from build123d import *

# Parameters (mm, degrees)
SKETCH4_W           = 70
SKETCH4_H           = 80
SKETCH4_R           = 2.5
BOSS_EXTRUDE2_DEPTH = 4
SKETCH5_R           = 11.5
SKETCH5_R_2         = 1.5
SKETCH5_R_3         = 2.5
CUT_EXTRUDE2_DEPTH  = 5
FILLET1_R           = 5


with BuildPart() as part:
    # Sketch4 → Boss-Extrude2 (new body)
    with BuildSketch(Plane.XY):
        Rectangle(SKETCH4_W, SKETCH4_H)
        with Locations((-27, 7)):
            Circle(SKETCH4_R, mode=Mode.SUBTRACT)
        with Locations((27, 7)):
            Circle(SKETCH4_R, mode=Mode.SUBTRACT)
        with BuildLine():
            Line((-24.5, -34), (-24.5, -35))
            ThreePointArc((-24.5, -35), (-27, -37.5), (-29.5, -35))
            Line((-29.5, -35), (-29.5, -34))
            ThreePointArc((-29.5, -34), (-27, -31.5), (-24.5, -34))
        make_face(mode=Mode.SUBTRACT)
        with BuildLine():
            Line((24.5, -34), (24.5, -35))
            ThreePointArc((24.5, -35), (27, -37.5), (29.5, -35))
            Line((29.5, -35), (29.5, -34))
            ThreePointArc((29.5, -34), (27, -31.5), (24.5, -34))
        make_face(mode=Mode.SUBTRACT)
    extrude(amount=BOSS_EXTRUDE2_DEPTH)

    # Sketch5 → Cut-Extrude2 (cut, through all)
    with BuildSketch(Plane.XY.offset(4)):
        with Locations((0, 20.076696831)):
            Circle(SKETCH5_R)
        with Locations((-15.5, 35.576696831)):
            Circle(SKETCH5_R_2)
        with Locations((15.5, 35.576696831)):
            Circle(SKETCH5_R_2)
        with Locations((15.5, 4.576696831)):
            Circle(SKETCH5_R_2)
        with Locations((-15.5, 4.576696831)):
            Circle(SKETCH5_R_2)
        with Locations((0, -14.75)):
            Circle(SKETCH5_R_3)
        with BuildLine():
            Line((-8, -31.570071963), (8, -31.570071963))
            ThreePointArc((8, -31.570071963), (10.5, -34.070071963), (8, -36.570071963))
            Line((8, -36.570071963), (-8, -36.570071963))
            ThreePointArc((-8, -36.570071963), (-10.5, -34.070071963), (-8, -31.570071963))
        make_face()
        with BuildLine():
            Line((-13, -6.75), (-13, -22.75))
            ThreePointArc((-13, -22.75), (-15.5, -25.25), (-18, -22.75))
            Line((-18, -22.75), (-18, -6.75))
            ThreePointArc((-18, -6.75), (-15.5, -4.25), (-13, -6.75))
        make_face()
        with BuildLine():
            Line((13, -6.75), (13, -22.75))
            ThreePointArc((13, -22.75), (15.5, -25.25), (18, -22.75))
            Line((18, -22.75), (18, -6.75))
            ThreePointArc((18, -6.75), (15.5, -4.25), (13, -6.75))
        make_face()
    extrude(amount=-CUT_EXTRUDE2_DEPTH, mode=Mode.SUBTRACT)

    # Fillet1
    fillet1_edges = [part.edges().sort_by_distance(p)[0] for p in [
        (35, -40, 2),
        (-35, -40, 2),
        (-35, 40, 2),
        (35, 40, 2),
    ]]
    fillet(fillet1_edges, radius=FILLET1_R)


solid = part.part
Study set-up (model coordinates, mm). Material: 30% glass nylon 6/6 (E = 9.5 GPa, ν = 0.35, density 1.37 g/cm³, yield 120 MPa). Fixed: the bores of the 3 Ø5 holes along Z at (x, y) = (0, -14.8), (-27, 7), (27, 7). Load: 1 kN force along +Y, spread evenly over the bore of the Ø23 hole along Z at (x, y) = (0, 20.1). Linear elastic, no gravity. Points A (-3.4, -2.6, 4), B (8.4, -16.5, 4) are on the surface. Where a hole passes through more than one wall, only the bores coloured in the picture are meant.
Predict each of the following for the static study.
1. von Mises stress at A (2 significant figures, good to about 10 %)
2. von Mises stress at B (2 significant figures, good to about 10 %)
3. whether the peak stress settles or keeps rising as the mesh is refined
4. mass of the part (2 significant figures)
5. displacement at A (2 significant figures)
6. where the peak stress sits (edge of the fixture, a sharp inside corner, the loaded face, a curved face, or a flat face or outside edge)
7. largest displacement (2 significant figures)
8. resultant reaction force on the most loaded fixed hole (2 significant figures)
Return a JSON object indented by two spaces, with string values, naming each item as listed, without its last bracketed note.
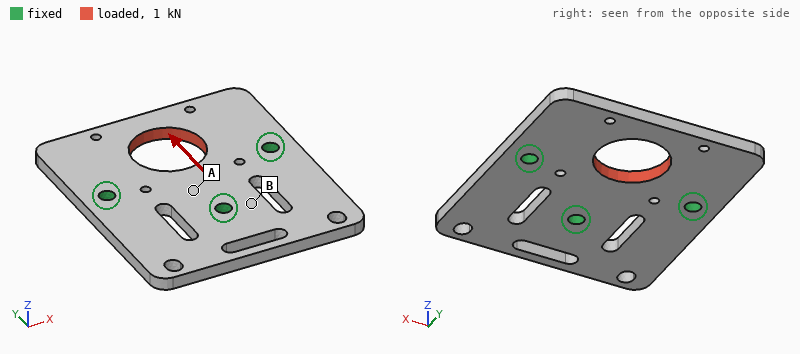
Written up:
{
  "von Mises stress at A": "4.6 MPa",
  "von Mises stress at B": "1.7 MPa",
  "whether the peak stress settles or keeps rising as the mesh is refined": "keeps rising",
  "mass of the part": "26 g",
  "displacement at A": "6.4 µm",
  "where the peak stress sits": "edge of the fixture",
  "largest displacement": "33 µm",
  "resultant reaction force on the most loaded fixed hole": "360 N"
}
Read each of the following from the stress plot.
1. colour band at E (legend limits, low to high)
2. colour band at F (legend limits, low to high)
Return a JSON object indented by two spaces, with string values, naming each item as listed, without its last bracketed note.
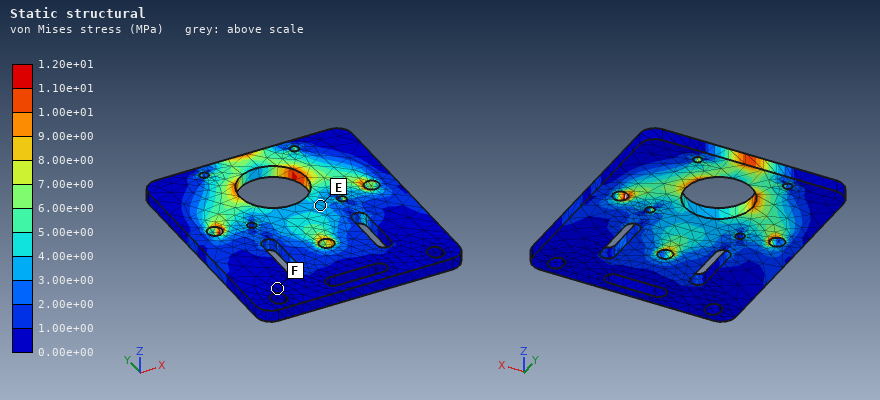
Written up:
{
  "colour band at E": "3.00e+00 to 4.00e+00 MPa",
  "colour band at F": "0.00e+00 to 1.00e+00 MPa"
}
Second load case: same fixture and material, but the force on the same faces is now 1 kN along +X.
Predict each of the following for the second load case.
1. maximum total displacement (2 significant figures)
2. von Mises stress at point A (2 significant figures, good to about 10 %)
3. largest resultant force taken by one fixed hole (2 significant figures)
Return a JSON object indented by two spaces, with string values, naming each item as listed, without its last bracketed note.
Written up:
{
  "maximum total displacement": "52 µm",
  "von Mises stress at point A": "3.3 MPa",
  "largest resultant force taken by one fixed hole": "510 N"
}
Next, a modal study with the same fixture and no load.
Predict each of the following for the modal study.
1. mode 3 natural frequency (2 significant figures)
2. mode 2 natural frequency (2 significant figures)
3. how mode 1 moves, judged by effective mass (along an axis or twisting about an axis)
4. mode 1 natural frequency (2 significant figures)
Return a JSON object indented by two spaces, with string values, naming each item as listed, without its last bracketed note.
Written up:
{
  "mode 3 natural frequency": "1600 Hz",
  "mode 2 natural frequency": "1600 Hz",
  "how mode 1 moves, judged by effective mass": "along Z",
  "mode 1 natural frequency": "1400 Hz"
}
